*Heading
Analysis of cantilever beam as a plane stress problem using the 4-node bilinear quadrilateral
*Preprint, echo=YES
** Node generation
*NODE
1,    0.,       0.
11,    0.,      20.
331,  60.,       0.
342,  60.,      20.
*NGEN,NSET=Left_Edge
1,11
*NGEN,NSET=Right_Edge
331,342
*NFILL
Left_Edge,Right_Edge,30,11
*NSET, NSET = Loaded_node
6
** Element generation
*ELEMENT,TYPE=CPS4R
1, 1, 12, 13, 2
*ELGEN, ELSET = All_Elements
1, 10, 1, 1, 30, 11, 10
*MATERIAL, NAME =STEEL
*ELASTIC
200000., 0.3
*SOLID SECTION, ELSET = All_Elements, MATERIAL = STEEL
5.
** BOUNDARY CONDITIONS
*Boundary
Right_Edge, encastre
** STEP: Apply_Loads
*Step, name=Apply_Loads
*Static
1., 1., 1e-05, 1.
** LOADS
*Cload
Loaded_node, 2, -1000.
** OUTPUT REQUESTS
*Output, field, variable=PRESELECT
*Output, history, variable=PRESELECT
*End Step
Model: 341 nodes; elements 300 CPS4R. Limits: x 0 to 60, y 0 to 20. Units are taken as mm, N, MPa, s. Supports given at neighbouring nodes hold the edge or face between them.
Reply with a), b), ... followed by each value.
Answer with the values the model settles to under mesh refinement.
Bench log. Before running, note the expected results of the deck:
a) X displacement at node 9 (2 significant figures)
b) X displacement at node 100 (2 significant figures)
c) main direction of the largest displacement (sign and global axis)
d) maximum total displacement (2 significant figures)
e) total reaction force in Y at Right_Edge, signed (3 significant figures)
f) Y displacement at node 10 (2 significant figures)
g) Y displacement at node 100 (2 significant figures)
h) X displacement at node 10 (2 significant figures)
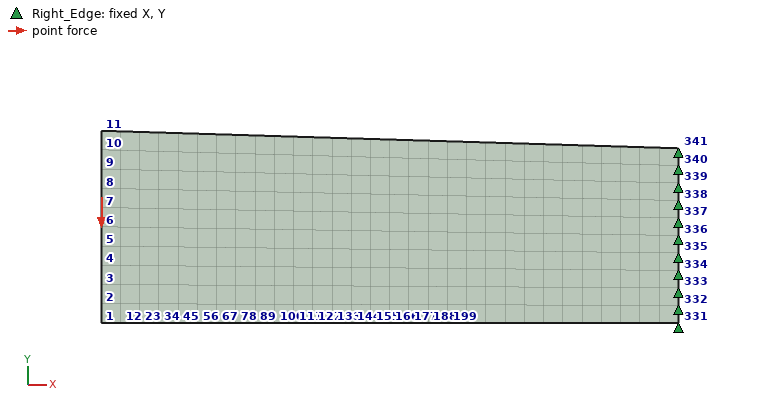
a) -0.022 mm
b) 0.028 mm
c) -Y
d) 0.15 mm
e) 1000 N
f) -0.14 mm
g) -0.083 mm
h) -0.028 mm
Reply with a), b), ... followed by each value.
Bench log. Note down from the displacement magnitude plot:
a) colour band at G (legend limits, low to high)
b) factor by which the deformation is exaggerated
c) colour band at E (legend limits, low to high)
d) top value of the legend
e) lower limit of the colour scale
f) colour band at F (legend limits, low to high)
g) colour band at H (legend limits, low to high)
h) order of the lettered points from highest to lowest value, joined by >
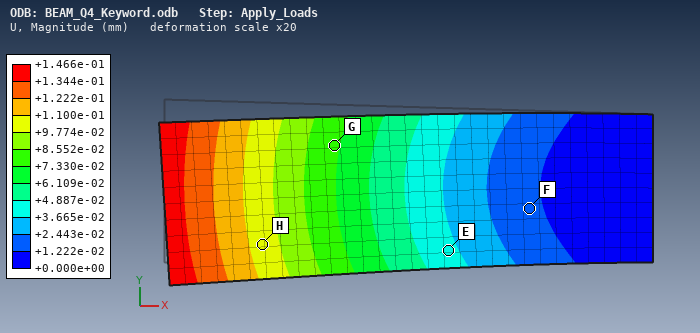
a) +7.330e-02 to +8.552e-02 mm
b) 20
c) +3.665e-02 to +4.887e-02 mm
d) +1.466e-01 mm
e) +0.000e+00 mm
f) +1.222e-02 to +2.443e-02 mm
g) +9.774e-02 to +1.100e-01 mm
h) H > G > E > F
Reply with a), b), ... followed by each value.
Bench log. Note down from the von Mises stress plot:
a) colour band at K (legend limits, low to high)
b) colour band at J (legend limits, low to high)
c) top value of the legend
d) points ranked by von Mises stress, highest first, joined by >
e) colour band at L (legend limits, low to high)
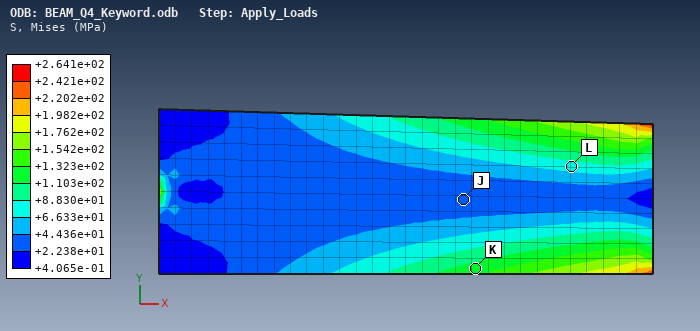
a) +1.103e+02 to +1.323e+02 MPa
b) +2.238e+01 to +4.436e+01 MPa
c) +2.641e+02 MPa
d) K > L > J
e) +6.633e+01 to +8.830e+01 MPa
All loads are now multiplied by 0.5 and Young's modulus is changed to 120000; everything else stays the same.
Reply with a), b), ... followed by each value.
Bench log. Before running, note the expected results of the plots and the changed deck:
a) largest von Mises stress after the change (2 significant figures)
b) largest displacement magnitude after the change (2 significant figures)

a) 130 MPa
b) 0.12 mm
